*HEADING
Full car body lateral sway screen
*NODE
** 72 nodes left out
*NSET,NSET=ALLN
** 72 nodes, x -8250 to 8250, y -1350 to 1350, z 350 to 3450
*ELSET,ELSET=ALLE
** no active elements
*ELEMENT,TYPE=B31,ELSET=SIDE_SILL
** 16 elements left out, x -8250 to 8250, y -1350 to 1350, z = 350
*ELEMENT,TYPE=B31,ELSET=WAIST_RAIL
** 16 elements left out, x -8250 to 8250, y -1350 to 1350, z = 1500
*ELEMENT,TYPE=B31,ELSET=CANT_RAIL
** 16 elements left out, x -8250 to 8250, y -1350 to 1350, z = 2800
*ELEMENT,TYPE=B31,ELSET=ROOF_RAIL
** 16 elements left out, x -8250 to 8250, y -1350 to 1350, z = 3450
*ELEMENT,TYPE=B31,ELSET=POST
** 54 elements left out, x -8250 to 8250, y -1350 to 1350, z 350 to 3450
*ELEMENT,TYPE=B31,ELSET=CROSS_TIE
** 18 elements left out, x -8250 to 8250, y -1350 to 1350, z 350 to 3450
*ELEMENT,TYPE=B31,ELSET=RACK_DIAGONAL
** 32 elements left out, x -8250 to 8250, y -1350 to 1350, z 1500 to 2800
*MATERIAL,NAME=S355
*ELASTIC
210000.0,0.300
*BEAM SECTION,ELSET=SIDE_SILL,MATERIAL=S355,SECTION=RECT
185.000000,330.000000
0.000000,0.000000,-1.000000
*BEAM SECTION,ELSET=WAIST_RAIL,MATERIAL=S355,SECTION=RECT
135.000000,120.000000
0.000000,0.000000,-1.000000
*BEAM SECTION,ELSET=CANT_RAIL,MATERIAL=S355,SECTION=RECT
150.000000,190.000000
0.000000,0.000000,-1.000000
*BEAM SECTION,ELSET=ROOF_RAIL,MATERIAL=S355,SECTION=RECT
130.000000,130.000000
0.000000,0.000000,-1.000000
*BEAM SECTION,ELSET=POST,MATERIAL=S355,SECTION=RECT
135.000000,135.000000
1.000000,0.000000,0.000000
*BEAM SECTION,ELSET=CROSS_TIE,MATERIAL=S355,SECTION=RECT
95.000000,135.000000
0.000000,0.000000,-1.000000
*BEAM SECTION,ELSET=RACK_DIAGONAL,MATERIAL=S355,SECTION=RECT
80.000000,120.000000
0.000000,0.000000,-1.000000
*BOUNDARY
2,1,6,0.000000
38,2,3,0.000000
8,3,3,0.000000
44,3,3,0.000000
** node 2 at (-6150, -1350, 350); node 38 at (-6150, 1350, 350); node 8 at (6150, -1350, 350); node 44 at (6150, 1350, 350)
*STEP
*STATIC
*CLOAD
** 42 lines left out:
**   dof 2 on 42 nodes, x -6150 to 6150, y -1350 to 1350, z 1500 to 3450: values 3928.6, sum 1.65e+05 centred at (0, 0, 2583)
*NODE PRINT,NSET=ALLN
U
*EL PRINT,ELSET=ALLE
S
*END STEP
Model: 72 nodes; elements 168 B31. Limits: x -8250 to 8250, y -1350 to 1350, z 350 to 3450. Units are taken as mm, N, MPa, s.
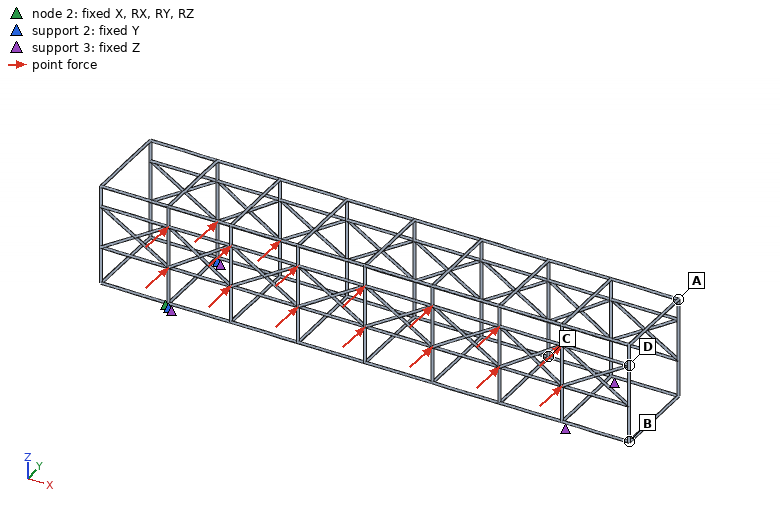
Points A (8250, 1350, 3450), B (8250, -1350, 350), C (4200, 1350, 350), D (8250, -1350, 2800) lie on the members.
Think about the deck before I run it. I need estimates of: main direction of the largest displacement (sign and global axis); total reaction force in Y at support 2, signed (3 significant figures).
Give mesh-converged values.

+Y
-1.65e+05 N
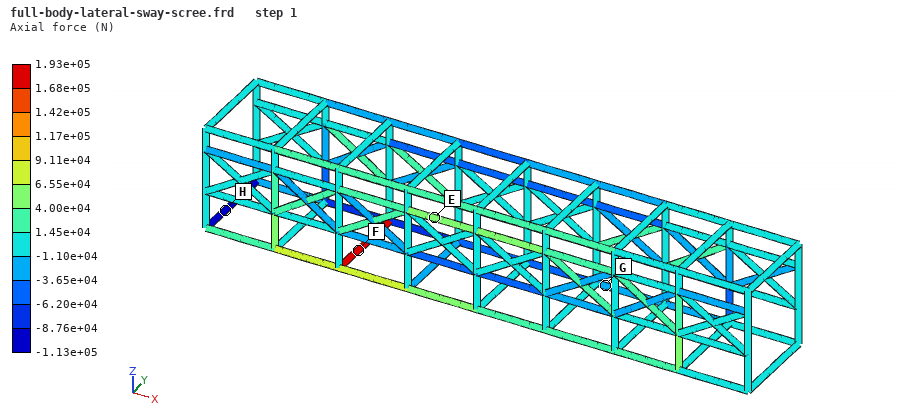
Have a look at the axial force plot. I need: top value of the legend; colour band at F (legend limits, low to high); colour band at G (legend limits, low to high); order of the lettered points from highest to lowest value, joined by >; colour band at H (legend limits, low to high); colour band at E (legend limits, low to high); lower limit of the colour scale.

1.93e+05 N
1.68e+05 to 1.93e+05 N
-3.65e+04 to -1.10e+04 N
F > E > G > H
-1.13e+05 to -8.76e+04 N
4.00e+04 to 6.55e+04 N
-1.13e+05 N
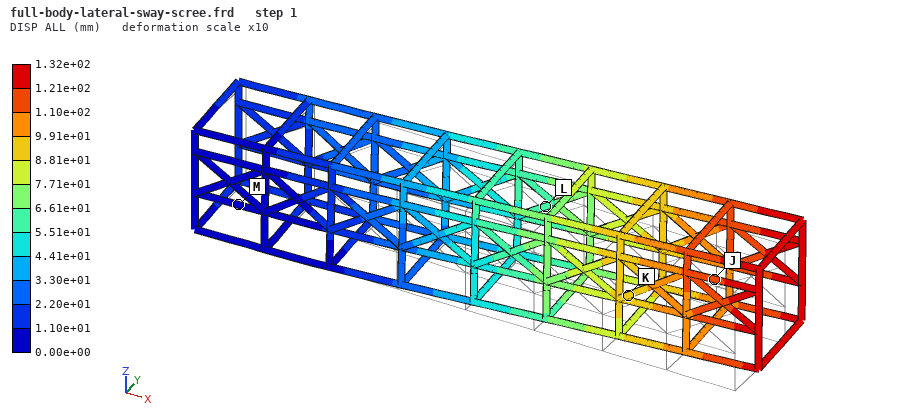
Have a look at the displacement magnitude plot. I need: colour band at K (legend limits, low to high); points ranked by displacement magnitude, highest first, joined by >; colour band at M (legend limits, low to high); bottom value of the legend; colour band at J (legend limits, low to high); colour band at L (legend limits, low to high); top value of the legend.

8.81e+01 to 9.91e+01 mm
J > K > L > M
0.00e+00 to 1.10e+01 mm
0.00e+00 mm
1.10e+02 to 1.21e+02 mm
5.51e+01 to 6.61e+01 mm
1.32e+02 mm
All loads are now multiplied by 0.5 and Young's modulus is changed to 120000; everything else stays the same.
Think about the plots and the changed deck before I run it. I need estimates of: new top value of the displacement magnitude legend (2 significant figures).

120 mm
